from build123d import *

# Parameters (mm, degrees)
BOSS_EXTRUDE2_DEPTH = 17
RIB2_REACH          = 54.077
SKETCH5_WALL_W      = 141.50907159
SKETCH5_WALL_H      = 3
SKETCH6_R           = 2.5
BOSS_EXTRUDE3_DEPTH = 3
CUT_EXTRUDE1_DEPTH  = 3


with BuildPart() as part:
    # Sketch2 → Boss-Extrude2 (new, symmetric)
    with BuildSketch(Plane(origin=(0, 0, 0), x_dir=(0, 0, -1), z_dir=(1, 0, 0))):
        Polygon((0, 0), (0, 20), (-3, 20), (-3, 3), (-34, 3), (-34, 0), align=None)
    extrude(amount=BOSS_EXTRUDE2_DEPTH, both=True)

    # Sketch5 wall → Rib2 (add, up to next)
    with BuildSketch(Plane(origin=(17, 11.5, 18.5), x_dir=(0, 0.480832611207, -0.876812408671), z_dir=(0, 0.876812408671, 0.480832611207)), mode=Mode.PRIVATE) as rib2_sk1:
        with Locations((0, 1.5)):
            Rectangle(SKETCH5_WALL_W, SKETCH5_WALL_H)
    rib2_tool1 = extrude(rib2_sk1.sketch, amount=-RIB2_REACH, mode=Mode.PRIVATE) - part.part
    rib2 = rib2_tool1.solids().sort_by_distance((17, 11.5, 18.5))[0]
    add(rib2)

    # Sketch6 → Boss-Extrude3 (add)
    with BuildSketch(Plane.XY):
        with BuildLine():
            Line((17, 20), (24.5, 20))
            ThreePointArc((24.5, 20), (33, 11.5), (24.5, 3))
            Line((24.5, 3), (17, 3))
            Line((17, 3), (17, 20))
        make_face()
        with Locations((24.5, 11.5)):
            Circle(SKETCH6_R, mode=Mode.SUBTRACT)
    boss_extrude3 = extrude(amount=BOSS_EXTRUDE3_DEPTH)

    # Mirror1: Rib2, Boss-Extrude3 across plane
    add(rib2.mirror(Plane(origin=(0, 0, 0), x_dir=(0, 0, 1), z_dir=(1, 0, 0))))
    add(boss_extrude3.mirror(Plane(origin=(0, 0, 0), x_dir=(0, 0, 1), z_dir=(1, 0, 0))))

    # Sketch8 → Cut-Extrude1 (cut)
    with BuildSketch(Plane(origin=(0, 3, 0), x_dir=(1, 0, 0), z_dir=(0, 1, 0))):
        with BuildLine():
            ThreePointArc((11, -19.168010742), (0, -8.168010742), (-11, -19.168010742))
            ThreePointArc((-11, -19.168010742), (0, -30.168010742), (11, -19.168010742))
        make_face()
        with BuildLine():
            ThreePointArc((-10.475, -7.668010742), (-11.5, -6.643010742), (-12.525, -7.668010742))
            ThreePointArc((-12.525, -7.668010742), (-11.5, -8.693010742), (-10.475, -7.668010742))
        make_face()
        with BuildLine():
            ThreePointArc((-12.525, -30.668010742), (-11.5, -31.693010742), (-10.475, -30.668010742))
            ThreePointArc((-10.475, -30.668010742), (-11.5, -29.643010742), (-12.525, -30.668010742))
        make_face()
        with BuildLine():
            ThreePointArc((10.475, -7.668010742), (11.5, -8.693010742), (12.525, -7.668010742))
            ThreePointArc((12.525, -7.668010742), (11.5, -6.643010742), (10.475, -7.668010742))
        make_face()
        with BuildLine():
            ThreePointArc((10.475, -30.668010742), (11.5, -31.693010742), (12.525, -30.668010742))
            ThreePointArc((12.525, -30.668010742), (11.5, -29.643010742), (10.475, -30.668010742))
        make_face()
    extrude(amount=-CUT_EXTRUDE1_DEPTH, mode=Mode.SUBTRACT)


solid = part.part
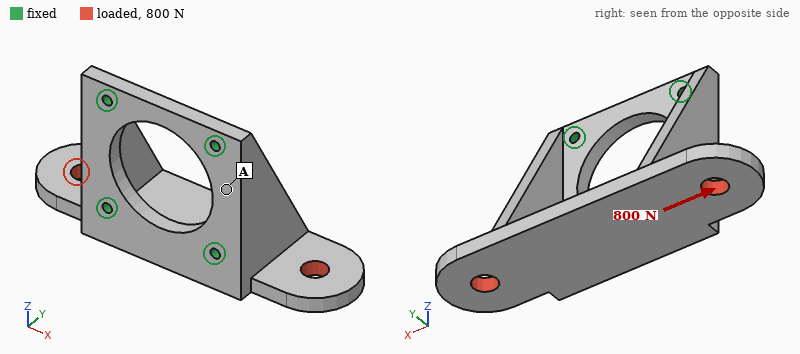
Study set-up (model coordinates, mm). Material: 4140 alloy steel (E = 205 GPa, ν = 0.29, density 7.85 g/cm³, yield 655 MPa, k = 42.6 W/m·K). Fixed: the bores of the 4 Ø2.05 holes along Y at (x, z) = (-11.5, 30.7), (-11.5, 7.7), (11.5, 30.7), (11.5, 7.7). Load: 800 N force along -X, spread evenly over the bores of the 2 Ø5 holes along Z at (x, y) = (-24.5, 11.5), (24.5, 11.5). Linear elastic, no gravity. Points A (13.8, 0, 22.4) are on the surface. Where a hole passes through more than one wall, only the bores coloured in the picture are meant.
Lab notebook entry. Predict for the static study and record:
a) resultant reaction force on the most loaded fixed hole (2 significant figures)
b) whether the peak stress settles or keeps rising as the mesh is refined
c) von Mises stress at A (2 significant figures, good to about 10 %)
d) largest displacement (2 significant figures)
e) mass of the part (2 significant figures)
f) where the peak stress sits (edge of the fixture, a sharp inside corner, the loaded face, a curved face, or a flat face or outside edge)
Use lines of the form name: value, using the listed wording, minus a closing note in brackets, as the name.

resultant reaction force on the most loaded fixed hole: 560 N
whether the peak stress settles or keeps rising as the mesh is refined: keeps rising
von Mises stress at A: 8.7 MPa
largest displacement: 8.4 µm
mass of the part: 54 g
where the peak stress sits: edge of the fixture
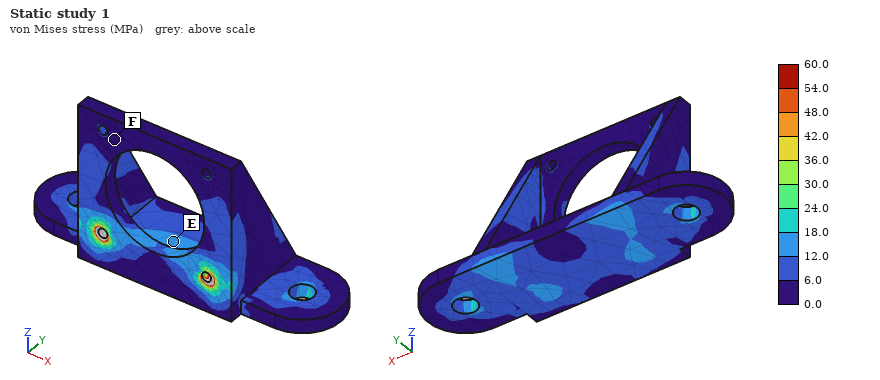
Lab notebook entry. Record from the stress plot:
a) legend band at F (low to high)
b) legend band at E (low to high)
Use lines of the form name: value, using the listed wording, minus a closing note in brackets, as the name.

legend band at F: 0.0 to 6.0 MPa
legend band at E: 12.0 to 18.0 MPa
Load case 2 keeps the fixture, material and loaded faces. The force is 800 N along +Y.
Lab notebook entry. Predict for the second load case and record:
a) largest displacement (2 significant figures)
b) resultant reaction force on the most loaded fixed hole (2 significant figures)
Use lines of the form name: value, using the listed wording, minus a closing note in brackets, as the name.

largest displacement: 8.5 µm
resultant reaction force on the most loaded fixed hole: 520 N
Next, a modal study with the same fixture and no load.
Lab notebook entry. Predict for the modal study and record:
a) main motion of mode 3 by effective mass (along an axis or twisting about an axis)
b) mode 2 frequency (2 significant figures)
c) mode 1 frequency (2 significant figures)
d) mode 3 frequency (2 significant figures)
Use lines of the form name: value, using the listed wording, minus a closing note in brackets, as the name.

main motion of mode 3 by effective mass: along X
mode 2 frequency: 7500 Hz
mode 1 frequency: 7400 Hz
mode 3 frequency: 9300 Hz
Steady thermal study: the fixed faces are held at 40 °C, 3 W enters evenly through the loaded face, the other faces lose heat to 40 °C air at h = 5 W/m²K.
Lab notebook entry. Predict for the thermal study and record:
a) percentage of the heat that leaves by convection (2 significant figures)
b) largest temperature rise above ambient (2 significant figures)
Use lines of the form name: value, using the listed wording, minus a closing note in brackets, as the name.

percentage of the heat that leaves by convection: 4.4 %
largest temperature rise above ambient: 15 K
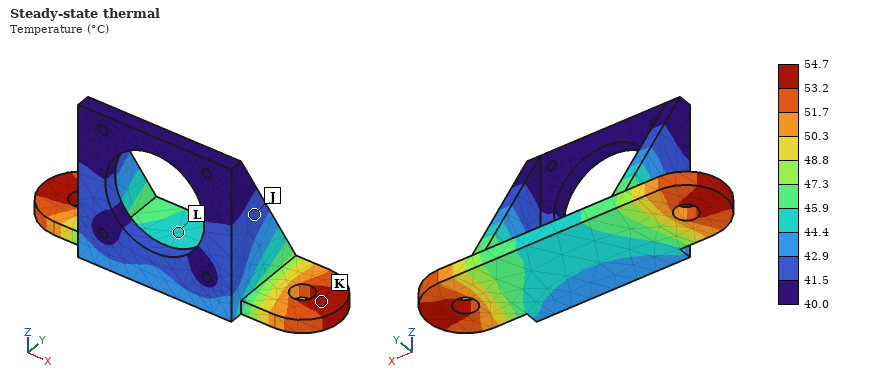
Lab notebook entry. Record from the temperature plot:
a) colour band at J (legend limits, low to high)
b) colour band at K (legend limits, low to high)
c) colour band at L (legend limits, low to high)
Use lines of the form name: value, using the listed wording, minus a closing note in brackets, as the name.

colour band at J: 41.5 to 42.9 °C
colour band at K: 53.2 to 54.7 °C
colour band at L: 44.4 to 45.9 °C
